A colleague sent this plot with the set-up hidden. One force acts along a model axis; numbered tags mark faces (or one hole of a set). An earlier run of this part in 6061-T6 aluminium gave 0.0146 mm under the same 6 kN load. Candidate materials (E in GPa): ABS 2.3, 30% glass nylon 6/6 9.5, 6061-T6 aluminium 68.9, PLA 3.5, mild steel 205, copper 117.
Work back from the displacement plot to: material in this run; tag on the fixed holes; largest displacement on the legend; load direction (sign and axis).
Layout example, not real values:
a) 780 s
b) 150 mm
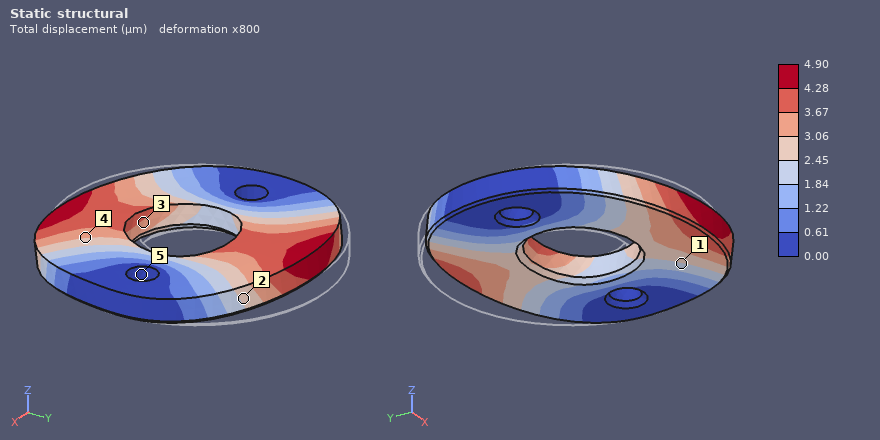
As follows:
a) mild steel
b) 5
c) 4.90 µm
d) -Y
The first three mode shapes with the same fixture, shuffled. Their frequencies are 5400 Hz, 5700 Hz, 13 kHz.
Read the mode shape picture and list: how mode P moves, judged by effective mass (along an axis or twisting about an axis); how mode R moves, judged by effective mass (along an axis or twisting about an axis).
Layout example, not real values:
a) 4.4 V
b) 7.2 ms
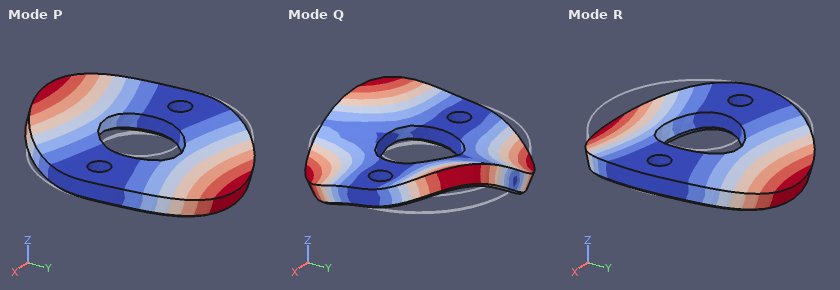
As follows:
a) twisting about X
b) along Z
